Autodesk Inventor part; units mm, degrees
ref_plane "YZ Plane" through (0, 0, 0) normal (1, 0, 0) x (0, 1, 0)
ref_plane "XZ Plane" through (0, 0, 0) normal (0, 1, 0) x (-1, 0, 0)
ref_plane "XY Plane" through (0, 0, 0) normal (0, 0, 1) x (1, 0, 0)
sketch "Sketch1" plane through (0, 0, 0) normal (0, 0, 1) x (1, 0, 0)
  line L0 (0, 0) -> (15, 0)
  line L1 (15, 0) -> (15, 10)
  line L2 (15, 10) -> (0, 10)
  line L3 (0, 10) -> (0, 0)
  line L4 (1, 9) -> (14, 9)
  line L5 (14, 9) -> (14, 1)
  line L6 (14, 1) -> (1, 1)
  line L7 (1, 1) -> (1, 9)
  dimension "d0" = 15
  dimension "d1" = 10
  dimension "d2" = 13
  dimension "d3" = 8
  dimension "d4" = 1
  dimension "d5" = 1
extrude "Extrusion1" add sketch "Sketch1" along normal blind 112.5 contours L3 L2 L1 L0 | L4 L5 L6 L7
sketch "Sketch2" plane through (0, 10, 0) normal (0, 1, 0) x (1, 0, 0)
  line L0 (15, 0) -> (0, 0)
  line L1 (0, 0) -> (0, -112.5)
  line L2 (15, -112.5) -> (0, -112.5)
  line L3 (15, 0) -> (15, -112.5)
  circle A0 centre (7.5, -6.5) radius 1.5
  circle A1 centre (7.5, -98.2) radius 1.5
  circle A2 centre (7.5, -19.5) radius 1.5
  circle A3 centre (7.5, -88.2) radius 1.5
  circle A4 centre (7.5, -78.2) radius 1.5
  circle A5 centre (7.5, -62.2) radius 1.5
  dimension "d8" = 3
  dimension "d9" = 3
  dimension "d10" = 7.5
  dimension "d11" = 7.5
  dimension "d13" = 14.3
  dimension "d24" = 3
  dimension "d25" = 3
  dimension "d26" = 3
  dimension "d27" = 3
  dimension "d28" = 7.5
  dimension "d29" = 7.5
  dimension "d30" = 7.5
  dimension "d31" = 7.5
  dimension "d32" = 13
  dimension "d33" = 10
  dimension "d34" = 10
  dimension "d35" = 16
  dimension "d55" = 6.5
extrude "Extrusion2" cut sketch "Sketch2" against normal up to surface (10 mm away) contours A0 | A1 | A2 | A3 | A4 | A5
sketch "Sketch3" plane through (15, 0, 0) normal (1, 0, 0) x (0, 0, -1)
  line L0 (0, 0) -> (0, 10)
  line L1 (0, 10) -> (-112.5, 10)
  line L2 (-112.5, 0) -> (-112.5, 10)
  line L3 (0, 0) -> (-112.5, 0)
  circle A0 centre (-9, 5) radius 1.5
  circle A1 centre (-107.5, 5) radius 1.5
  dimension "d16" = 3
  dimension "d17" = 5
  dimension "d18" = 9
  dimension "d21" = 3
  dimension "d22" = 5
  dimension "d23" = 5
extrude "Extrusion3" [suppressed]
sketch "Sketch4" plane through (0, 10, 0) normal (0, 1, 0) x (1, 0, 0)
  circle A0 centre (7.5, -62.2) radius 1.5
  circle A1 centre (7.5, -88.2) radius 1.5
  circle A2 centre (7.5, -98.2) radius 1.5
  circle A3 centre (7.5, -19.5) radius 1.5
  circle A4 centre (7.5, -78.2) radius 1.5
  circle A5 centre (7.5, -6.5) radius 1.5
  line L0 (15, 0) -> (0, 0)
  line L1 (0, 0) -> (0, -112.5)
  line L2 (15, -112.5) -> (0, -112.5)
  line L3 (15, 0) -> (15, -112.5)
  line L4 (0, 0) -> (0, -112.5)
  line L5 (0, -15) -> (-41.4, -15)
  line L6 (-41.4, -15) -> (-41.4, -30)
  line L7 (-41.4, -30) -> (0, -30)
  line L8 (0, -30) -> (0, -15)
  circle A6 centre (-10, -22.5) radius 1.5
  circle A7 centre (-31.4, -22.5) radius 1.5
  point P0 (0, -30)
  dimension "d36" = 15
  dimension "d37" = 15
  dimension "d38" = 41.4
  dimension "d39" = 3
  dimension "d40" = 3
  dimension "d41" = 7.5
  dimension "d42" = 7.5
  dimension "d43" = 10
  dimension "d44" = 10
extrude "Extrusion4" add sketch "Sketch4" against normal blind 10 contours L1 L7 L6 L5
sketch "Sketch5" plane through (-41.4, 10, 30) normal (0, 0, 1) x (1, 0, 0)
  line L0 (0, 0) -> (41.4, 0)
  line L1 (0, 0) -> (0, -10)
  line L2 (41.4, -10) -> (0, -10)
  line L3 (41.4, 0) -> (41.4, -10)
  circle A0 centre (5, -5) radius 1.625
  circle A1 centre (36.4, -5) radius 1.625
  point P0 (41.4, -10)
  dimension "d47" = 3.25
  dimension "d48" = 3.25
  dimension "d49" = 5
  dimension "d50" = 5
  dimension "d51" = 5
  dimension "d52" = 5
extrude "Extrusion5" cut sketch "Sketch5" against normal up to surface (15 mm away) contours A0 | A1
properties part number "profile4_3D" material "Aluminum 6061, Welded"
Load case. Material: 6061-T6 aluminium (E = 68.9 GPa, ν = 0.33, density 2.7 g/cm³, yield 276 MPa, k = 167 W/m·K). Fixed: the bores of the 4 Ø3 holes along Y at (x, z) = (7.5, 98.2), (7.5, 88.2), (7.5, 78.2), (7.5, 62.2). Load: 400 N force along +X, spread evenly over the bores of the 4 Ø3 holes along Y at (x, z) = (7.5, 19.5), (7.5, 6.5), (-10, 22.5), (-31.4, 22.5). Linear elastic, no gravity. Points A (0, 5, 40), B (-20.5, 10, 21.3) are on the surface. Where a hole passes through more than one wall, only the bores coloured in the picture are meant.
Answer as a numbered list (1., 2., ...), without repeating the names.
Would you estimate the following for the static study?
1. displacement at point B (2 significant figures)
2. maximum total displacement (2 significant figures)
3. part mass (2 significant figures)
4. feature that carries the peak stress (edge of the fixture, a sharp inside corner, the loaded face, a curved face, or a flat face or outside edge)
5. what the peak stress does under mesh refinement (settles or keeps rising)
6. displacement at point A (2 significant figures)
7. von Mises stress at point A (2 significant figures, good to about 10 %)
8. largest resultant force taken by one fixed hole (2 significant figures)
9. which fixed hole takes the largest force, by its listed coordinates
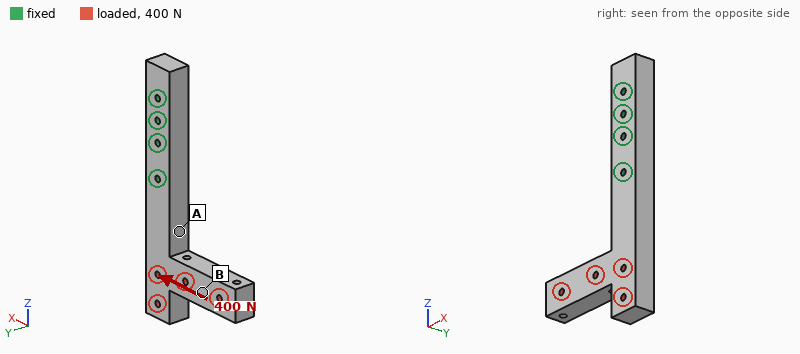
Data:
1. 0.11 mm
2. 0.16 mm
3. 60 g
4. edge of the fixture
5. keeps rising
6. 0.039 mm
7. 24 MPa
8. 1.2 kN
9. (7.5, 62.2)
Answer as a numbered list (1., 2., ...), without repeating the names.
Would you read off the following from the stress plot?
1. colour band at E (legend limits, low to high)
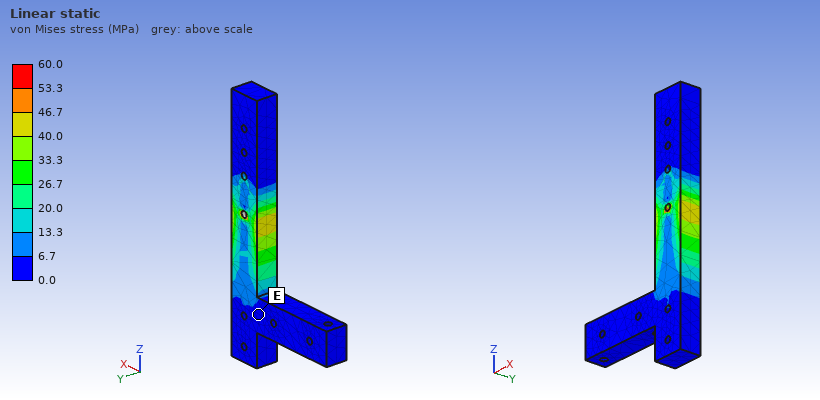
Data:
1. 0.0 to 6.7 MPa
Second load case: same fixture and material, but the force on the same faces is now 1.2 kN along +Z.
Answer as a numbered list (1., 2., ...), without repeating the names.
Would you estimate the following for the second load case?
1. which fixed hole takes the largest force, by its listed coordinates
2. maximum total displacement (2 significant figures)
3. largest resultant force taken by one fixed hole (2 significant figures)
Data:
1. (7.5, 62.2)
2. 0.27 mm
3. 1.2 kN
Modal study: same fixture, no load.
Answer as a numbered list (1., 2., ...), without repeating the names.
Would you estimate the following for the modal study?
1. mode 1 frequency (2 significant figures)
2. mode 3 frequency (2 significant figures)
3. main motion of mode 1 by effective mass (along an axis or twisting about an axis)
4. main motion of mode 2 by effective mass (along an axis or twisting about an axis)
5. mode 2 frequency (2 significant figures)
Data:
1. 1300 Hz
2. 2400 Hz
3. along Y
4. along X
5. 1600 Hz
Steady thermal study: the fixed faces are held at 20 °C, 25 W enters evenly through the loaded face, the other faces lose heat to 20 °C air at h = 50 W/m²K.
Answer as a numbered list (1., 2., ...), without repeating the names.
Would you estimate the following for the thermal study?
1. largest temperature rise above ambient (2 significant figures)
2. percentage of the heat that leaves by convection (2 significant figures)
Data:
1. 37 K
2. 30 %
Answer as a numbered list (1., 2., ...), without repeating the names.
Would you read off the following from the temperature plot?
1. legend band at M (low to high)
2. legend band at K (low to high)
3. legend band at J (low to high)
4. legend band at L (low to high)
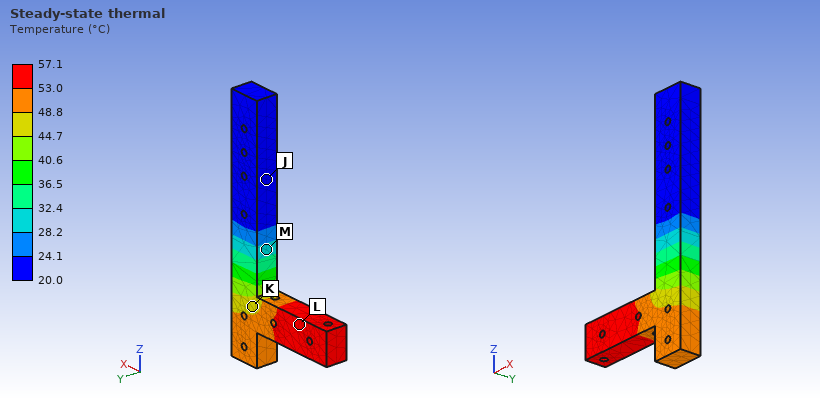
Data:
1. 28.2 to 32.4 °C
2. 44.7 to 48.8 °C
3. 20.0 to 24.1 °C
4. 53.0 to 57.1 °C
